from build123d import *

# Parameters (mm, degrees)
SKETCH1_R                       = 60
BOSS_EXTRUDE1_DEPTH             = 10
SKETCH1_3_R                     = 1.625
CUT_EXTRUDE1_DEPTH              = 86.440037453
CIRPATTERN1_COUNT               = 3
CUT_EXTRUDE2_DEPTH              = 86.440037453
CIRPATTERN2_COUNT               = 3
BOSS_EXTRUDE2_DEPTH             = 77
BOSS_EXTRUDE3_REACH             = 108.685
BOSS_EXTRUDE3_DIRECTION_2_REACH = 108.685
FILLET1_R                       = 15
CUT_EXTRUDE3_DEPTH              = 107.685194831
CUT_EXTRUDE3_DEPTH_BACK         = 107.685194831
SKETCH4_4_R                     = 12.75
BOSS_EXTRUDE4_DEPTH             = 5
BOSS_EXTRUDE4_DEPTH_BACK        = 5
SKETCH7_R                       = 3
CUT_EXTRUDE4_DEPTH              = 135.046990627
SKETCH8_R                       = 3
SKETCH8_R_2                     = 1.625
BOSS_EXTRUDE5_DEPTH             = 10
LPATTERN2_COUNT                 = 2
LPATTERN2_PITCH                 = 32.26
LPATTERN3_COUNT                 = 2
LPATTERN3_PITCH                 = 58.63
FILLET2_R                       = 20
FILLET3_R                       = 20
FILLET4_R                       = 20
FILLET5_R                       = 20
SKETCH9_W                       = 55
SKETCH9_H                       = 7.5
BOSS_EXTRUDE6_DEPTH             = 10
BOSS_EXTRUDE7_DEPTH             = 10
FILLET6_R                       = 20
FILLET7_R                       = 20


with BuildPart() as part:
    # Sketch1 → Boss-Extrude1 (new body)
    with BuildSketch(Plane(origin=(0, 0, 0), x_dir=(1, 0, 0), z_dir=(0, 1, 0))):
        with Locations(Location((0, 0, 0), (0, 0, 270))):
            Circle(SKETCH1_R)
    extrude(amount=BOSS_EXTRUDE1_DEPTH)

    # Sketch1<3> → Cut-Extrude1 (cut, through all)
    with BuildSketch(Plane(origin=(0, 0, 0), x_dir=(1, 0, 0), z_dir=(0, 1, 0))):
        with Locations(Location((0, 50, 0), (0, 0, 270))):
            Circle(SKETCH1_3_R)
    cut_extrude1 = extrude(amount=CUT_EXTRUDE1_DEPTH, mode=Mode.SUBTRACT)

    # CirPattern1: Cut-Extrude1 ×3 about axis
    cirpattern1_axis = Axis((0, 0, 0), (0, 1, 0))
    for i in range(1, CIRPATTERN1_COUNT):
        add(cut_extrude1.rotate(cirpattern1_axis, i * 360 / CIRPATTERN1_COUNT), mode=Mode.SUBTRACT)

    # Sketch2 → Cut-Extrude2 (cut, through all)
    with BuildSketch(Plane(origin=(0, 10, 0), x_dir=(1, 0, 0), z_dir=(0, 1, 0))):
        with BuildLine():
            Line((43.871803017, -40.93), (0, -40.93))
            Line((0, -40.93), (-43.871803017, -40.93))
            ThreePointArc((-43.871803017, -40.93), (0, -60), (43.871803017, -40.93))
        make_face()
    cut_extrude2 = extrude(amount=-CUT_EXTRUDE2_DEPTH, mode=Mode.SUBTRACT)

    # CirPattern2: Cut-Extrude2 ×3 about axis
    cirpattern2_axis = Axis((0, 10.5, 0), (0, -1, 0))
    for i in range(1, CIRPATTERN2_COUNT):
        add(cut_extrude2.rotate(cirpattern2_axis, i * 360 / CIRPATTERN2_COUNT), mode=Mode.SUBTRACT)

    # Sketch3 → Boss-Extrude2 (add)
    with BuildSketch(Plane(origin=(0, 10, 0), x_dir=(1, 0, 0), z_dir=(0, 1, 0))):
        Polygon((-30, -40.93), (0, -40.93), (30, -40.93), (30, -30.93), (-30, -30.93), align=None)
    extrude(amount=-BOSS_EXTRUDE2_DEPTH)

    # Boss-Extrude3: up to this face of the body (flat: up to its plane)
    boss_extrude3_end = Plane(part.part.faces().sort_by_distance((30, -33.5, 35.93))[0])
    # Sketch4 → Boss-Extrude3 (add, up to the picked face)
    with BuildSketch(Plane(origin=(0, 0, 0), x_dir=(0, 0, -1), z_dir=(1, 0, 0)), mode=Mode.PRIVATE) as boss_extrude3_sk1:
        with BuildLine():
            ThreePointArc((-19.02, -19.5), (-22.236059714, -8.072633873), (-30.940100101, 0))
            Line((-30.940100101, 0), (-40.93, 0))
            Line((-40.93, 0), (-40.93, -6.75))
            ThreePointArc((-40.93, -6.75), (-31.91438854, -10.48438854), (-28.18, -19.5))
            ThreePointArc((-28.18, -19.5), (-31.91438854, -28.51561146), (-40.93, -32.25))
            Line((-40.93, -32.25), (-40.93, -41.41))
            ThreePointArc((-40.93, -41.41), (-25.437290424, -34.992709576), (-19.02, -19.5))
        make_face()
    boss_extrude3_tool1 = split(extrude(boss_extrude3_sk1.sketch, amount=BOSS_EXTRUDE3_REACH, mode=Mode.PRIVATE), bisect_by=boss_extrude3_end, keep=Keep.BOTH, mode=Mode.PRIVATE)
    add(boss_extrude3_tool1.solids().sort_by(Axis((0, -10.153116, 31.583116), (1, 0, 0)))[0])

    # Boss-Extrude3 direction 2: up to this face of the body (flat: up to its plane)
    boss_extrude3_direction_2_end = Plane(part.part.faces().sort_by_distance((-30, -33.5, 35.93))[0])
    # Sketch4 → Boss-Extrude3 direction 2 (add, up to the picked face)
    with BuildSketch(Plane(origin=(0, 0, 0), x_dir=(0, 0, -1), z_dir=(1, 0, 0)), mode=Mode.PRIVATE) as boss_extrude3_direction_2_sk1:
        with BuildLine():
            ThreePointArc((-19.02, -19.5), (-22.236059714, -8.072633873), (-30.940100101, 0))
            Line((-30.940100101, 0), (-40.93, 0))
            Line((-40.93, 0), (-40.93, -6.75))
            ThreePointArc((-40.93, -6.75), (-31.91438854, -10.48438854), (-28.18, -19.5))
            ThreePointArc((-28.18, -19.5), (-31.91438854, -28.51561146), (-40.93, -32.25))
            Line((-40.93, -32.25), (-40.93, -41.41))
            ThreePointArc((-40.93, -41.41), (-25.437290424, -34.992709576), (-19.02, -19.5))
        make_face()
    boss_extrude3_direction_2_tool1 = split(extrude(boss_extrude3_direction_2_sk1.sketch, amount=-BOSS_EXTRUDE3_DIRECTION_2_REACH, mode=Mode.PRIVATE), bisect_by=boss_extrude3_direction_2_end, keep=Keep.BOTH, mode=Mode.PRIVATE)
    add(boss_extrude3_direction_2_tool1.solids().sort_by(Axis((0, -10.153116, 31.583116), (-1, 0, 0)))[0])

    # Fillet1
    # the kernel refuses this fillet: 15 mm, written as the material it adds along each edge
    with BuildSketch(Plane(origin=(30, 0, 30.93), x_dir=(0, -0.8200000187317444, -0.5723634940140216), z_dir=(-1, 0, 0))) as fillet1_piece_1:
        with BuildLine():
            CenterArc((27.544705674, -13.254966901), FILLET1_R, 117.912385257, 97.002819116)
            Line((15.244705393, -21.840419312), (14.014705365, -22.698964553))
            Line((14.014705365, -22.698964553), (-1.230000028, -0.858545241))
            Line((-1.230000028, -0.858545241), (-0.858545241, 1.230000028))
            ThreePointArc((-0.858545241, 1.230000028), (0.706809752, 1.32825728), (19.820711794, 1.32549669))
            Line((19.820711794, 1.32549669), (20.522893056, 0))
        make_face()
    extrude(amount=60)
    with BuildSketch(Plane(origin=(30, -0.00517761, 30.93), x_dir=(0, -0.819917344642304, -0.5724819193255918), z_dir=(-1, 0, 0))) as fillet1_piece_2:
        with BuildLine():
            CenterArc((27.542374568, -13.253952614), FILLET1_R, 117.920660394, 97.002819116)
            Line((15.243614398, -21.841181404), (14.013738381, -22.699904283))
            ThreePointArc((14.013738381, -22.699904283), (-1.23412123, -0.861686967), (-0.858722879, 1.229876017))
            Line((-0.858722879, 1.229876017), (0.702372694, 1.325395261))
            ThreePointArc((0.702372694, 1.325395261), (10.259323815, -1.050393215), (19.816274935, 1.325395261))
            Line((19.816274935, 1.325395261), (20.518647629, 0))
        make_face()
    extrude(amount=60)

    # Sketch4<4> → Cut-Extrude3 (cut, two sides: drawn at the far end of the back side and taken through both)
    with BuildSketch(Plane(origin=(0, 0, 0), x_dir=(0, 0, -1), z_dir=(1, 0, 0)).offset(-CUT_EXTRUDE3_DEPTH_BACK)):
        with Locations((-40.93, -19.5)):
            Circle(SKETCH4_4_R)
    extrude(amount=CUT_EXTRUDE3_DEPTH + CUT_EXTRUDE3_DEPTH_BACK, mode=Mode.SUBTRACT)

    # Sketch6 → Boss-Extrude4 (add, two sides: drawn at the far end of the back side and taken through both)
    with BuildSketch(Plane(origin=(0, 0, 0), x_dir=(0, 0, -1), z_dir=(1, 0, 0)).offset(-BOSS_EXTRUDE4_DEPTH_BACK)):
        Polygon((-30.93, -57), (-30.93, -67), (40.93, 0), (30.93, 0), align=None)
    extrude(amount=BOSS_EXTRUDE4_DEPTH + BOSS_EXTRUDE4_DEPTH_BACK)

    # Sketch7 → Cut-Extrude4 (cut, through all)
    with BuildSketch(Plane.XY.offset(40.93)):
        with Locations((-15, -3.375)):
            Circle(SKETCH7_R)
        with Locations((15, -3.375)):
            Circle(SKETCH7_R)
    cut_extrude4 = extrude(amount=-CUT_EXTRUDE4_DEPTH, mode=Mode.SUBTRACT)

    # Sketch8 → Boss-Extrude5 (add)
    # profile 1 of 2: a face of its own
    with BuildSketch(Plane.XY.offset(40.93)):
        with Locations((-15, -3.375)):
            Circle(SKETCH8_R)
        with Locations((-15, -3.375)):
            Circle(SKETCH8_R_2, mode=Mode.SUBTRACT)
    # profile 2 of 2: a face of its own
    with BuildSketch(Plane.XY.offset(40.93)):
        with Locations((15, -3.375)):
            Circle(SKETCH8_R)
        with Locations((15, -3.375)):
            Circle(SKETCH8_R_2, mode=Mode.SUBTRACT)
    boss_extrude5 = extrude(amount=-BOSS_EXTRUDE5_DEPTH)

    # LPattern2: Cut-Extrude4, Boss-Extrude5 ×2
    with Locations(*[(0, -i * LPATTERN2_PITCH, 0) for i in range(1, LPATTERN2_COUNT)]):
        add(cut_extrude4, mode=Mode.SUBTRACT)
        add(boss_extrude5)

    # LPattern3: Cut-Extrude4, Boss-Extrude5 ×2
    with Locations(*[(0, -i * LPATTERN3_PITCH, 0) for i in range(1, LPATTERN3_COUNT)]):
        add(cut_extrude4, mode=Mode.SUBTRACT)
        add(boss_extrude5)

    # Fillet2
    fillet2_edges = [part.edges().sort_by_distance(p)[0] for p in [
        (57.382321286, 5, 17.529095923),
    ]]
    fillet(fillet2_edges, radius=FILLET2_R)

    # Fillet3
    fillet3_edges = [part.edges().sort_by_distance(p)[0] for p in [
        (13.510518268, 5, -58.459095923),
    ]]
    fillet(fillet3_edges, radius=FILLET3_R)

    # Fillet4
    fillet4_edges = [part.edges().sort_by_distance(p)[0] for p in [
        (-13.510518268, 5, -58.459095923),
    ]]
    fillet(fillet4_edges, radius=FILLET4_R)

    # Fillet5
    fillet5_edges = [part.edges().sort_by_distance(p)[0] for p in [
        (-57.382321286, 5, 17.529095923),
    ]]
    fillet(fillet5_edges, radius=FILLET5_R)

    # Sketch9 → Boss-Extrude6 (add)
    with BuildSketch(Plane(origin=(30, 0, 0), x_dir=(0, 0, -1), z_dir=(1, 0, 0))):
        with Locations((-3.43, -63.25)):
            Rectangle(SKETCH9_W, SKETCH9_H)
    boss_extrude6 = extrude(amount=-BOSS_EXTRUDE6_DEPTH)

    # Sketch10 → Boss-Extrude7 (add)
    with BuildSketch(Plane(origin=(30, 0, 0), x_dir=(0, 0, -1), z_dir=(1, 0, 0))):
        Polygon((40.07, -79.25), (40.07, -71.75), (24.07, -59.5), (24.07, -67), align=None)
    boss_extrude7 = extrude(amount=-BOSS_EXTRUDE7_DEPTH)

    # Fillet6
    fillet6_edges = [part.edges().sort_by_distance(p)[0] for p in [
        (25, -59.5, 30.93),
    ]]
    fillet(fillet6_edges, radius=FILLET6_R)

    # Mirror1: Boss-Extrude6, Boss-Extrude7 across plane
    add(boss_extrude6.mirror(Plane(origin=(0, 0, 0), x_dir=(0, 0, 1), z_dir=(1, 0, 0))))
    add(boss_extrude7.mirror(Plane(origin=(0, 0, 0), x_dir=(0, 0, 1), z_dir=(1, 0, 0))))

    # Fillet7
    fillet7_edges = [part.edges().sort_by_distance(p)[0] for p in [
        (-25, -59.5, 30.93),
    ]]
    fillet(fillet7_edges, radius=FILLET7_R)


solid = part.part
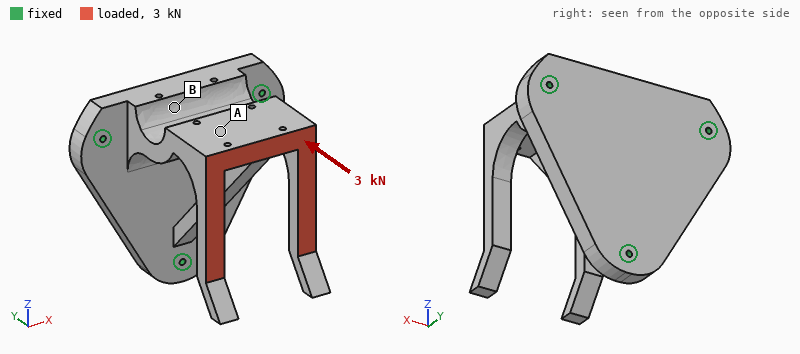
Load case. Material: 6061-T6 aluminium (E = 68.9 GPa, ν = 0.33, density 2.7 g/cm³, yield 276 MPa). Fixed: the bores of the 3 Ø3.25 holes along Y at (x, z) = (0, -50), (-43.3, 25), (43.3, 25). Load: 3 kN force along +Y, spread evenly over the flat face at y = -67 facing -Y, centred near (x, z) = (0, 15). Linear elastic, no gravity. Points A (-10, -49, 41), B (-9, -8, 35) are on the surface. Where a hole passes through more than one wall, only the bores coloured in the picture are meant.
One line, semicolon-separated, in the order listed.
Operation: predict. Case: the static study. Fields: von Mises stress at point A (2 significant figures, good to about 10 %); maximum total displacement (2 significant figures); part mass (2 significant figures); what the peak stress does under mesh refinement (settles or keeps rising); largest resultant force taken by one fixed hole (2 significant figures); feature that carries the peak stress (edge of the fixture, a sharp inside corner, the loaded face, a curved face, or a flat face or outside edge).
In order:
25 MPa; 0.93 mm; 390 g; keeps rising; 1.3 kN; edge of the fixture
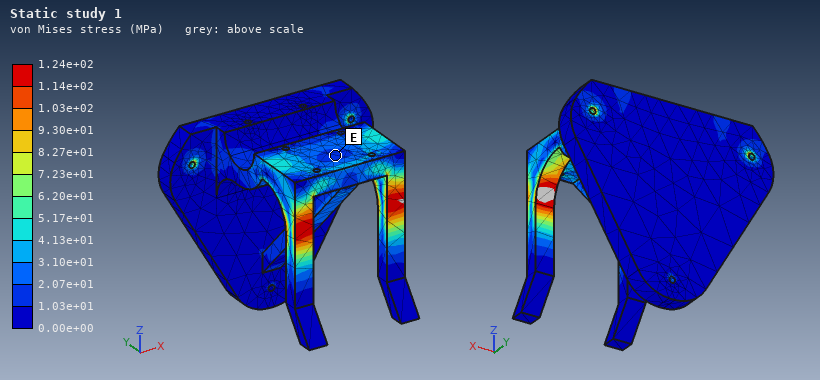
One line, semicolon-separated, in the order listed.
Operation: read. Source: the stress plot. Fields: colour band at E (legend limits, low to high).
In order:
1.03e+01 to 2.07e+01 MPa
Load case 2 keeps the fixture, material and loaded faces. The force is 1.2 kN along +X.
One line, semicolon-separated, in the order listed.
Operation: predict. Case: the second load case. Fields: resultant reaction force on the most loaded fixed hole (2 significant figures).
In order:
1.2 kN
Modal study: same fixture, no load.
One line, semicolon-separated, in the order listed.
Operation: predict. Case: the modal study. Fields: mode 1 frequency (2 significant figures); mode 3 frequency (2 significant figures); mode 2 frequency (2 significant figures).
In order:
1200 Hz; 1400 Hz; 1300 Hz
